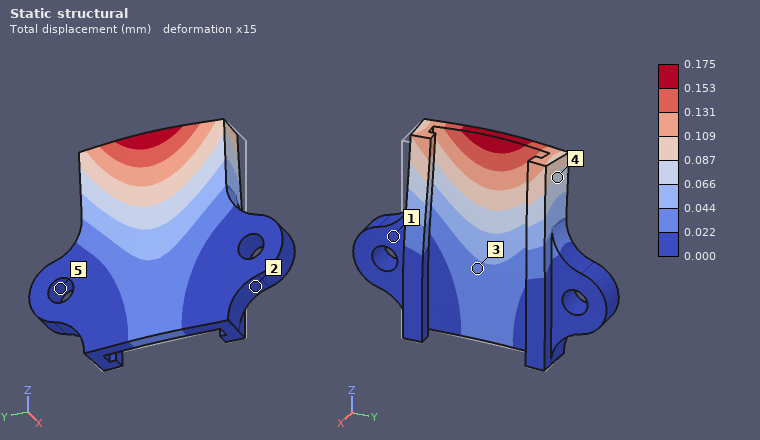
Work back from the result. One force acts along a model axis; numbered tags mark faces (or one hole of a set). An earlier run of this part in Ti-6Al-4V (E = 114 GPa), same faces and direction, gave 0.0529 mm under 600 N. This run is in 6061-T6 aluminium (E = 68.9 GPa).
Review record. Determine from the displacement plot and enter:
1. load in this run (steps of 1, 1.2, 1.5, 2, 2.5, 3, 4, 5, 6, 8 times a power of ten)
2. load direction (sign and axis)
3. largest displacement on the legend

1.2 kN
-X
0.175 mm
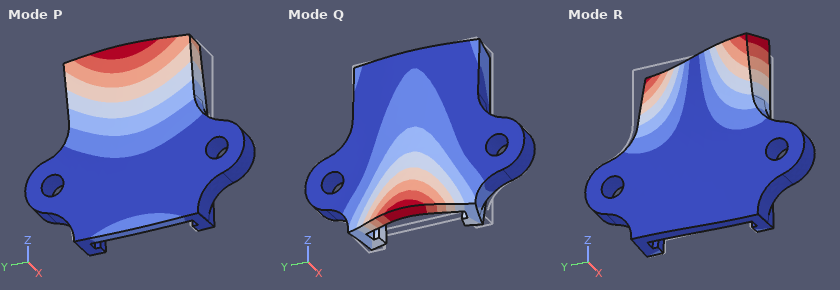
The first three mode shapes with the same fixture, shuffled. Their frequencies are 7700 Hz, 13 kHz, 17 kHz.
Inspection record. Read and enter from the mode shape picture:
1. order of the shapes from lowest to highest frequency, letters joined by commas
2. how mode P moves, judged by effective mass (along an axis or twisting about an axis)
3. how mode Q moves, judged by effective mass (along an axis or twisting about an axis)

P, R, Q
along X
along X
